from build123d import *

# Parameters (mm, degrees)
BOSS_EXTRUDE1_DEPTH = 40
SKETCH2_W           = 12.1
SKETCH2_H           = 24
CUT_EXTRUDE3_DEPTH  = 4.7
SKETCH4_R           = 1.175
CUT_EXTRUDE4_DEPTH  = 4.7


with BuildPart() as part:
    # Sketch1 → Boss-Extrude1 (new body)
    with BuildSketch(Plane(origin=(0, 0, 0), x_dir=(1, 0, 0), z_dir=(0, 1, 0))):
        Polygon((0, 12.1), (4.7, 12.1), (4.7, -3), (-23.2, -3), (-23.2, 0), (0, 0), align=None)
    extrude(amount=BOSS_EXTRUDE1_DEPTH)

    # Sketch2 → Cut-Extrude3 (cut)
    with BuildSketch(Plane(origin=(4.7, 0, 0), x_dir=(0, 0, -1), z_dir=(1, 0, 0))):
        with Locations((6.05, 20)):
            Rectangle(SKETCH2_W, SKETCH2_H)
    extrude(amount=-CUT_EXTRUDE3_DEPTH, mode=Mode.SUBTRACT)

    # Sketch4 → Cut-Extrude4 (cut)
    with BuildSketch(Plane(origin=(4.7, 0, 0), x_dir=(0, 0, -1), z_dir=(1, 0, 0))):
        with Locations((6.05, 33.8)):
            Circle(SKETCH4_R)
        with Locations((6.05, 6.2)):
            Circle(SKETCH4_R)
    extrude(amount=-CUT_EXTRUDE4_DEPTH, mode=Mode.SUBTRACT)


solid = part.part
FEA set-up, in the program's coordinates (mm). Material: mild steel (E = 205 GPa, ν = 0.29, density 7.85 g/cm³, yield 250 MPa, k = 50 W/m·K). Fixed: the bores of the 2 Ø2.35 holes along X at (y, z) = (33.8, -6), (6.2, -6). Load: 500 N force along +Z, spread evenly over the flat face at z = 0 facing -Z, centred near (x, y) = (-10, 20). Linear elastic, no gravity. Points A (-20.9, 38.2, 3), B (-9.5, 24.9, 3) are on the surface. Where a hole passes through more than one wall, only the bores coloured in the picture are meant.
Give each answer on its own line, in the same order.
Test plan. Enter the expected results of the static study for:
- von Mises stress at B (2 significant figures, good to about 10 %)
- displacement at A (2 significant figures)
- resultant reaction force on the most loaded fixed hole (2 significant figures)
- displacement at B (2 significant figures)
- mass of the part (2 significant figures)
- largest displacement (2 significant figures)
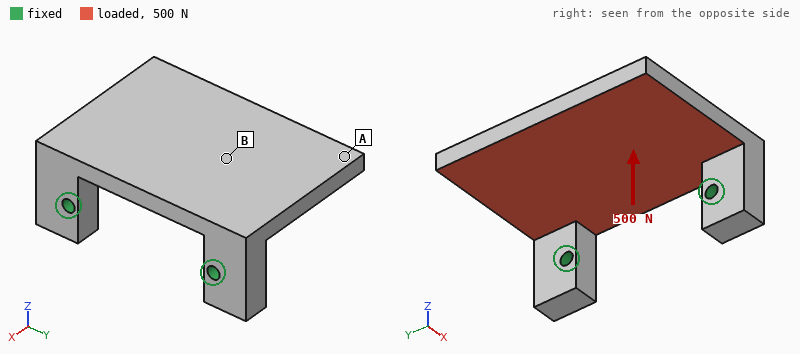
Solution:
33 MPa
0.095 mm
260 N
0.048 mm
33 g
0.11 mm
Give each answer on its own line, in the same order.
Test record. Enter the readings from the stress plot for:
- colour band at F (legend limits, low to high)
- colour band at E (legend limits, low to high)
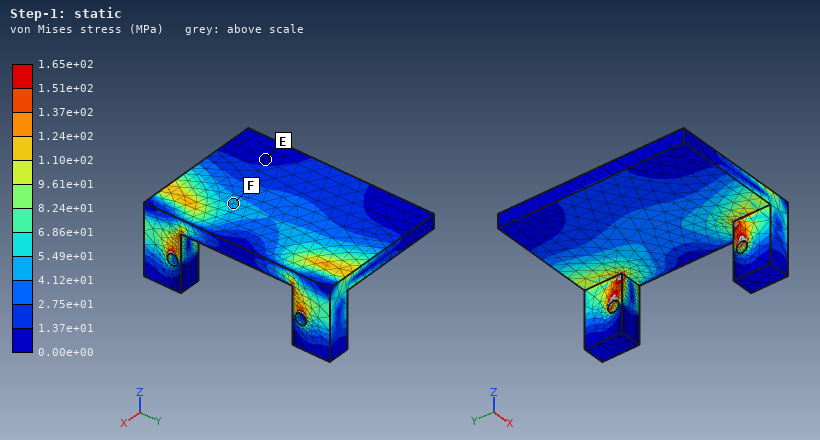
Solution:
4.12e+01 to 5.49e+01 MPa
0.00e+00 to 1.37e+01 MPa
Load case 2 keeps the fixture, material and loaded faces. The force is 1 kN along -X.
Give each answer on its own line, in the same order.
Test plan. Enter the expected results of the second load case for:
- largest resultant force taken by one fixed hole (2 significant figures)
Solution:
500 N
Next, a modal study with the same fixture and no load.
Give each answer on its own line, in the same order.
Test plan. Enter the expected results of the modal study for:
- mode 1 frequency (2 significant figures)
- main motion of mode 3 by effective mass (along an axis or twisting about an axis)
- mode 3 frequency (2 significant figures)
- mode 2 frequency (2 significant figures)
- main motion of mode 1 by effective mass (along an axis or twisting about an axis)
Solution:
2600 Hz
along Y
9400 Hz
6100 Hz
along Z
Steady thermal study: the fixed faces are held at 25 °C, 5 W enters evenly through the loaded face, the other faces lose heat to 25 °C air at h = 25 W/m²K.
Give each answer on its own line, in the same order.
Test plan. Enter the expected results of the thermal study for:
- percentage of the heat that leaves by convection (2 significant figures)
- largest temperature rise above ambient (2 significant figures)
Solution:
13 %
20 K
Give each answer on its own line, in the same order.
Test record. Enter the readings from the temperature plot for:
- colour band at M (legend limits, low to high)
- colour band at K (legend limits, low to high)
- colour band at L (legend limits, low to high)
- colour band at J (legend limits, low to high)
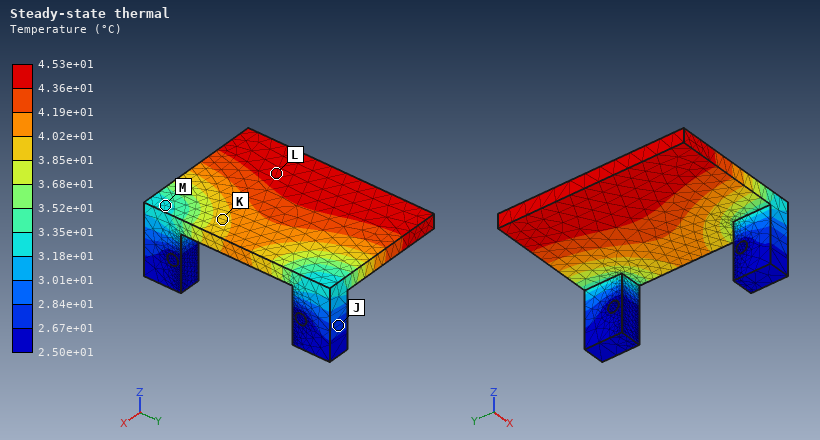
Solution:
3.18e+01 to 3.35e+01 °C
3.85e+01 to 4.02e+01 °C
4.36e+01 to 4.53e+01 °C
2.67e+01 to 2.84e+01 °C
